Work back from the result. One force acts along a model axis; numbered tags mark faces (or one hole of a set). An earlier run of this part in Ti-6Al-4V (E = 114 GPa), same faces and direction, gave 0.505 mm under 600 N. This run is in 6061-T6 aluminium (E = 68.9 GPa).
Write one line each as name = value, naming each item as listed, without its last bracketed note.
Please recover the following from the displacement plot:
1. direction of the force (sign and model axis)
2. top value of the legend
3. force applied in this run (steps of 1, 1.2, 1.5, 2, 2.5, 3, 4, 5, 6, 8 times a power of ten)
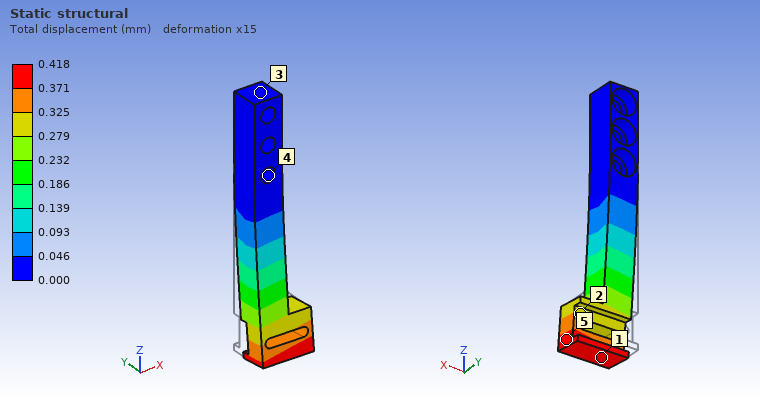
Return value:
direction of the force = -Y
top value of the legend = 0.418 mm
force applied in this run = 300 N
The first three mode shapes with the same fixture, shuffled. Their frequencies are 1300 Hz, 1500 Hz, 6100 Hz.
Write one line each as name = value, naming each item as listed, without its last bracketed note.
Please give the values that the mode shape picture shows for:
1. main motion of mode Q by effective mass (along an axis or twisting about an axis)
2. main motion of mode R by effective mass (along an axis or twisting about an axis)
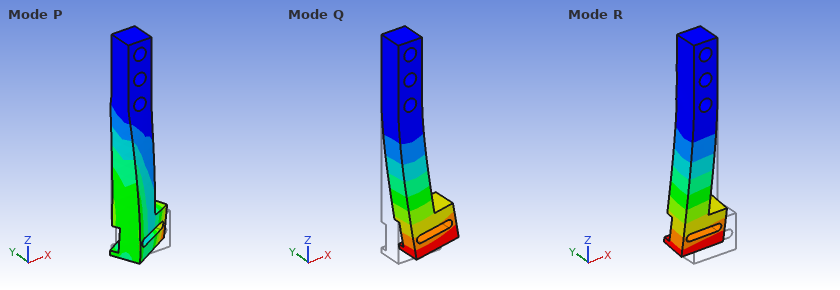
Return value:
main motion of mode Q by effective mass = along X
main motion of mode R by effective mass = along Y
